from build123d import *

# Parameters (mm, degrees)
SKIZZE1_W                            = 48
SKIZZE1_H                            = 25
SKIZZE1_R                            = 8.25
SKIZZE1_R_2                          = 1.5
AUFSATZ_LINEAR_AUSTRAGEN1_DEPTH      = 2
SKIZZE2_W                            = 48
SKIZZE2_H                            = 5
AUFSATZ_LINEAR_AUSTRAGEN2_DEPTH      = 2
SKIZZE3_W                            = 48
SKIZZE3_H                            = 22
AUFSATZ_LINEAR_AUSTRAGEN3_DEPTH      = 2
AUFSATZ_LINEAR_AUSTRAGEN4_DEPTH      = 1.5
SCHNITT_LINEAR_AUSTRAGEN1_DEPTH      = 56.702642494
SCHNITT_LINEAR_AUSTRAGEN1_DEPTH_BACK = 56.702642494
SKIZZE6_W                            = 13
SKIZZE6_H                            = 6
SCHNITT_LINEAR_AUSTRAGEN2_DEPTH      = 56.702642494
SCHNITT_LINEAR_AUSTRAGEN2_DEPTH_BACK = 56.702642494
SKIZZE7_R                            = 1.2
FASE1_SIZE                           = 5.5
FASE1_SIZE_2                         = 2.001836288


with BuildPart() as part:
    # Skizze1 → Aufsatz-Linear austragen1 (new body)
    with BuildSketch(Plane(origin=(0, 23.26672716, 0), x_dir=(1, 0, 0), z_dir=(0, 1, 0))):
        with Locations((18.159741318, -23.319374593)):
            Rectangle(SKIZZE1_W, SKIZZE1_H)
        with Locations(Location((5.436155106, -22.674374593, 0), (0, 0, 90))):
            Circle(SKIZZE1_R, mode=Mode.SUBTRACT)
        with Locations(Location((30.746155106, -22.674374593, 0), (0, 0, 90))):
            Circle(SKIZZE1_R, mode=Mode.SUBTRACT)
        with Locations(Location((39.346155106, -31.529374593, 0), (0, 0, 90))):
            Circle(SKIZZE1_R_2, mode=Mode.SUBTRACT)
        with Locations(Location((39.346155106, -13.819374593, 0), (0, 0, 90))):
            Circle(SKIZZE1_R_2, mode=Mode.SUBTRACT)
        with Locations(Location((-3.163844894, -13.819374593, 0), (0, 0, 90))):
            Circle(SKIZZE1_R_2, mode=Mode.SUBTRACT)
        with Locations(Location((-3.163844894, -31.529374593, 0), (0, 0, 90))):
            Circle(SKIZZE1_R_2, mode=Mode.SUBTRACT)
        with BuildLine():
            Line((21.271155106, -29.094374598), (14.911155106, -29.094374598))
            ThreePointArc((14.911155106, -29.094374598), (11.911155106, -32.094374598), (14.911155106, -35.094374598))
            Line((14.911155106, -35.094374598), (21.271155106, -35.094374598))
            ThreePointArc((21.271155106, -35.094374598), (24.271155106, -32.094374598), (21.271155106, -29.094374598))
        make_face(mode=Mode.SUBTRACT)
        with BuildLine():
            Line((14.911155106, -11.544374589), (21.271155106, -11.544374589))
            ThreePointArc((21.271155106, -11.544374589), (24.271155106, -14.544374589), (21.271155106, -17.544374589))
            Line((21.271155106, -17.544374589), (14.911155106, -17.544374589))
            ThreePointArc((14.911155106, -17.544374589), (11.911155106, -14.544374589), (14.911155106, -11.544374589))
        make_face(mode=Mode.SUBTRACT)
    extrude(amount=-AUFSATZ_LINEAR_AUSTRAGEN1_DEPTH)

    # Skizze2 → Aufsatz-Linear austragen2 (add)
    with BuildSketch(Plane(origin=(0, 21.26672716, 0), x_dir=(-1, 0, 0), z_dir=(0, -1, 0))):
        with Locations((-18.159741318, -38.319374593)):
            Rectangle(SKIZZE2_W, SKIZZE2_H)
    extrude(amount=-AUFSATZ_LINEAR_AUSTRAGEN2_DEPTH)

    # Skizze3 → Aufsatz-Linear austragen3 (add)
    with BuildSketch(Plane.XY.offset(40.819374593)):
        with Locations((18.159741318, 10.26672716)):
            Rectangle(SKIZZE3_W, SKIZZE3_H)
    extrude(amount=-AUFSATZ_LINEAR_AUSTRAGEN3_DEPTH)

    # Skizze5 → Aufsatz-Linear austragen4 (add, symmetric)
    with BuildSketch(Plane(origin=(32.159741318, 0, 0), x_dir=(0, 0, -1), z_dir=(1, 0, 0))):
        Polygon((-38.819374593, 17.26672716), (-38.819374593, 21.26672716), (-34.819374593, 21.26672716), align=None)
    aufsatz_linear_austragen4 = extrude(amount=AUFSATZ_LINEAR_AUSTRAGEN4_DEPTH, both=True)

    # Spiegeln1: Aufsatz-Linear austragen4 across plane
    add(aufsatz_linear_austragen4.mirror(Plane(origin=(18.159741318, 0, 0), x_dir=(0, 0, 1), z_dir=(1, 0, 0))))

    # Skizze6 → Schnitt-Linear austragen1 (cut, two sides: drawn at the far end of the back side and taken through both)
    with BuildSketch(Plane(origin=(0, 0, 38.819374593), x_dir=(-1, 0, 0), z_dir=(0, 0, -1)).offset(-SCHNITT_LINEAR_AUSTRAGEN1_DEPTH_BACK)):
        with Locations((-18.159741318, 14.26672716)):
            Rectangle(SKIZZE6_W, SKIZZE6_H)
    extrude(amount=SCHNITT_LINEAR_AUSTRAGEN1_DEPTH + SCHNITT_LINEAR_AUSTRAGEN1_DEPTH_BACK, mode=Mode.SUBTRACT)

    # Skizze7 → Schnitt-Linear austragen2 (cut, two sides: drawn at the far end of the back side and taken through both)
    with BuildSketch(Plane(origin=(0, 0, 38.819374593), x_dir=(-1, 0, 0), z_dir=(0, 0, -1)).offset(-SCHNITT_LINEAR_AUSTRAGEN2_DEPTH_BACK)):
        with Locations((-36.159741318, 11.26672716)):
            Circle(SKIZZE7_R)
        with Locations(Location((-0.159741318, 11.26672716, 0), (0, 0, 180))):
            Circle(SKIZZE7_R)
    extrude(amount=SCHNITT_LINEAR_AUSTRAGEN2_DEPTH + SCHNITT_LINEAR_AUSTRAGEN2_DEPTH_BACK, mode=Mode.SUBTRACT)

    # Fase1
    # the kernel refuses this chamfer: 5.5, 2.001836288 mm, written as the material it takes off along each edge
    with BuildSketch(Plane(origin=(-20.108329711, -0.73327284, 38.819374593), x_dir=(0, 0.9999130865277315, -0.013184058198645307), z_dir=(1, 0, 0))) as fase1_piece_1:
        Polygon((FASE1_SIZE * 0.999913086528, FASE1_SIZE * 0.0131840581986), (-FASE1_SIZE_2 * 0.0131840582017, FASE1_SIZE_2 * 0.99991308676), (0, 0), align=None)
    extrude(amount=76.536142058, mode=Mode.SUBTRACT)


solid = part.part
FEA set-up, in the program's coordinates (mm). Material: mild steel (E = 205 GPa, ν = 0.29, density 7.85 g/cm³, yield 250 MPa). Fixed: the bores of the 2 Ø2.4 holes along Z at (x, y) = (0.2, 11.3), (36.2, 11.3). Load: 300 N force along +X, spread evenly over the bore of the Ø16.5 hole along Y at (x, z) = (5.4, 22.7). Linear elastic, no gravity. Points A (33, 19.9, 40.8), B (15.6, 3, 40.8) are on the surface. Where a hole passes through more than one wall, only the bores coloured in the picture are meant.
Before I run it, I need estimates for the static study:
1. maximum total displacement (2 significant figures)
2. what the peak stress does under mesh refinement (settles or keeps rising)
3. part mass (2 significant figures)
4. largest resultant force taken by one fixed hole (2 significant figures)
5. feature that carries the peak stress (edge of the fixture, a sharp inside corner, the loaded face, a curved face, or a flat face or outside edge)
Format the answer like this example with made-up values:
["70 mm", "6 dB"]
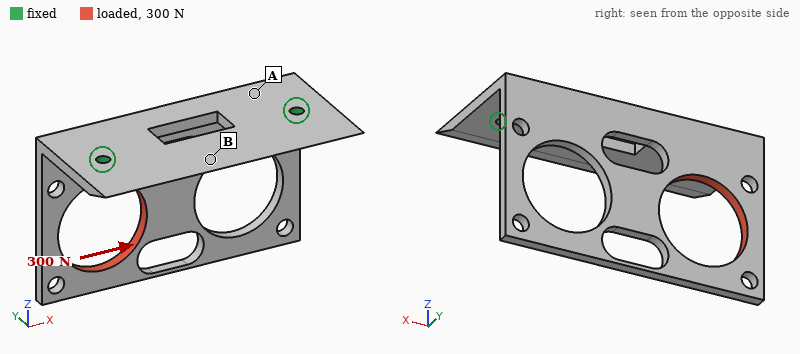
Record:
["59 µm", "keeps rising", "27 g", "220 N", "edge of the fixture"]
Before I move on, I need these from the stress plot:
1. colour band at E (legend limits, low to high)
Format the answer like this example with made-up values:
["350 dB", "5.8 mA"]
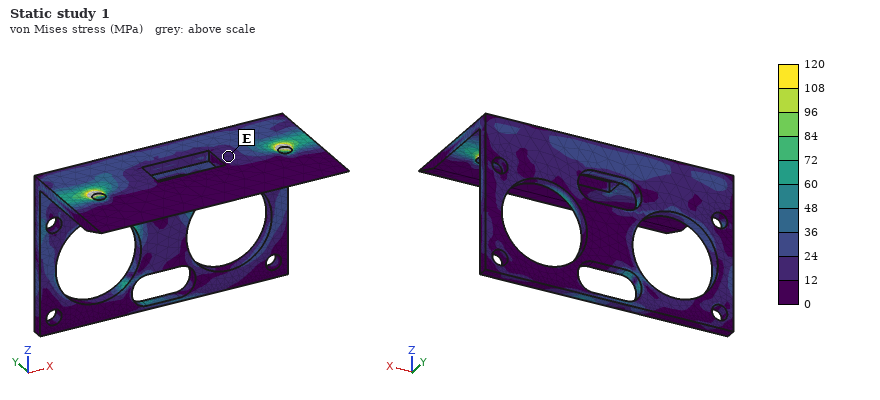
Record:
["12 to 24 MPa"]
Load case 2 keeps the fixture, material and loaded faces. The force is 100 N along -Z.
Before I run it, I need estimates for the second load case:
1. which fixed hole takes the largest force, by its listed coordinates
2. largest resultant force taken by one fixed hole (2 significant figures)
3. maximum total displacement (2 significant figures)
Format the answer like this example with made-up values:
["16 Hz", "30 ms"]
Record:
["(0.2, 11.3)", "84 N", "53 µm"]
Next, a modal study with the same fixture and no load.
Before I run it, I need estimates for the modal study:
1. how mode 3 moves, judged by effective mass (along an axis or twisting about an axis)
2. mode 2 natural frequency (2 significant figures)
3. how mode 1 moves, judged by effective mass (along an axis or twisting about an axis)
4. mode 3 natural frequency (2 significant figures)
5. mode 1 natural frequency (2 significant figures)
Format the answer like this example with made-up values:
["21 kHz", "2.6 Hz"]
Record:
["along Z", "2500 Hz", "along Y", "4500 Hz", "1400 Hz"]
